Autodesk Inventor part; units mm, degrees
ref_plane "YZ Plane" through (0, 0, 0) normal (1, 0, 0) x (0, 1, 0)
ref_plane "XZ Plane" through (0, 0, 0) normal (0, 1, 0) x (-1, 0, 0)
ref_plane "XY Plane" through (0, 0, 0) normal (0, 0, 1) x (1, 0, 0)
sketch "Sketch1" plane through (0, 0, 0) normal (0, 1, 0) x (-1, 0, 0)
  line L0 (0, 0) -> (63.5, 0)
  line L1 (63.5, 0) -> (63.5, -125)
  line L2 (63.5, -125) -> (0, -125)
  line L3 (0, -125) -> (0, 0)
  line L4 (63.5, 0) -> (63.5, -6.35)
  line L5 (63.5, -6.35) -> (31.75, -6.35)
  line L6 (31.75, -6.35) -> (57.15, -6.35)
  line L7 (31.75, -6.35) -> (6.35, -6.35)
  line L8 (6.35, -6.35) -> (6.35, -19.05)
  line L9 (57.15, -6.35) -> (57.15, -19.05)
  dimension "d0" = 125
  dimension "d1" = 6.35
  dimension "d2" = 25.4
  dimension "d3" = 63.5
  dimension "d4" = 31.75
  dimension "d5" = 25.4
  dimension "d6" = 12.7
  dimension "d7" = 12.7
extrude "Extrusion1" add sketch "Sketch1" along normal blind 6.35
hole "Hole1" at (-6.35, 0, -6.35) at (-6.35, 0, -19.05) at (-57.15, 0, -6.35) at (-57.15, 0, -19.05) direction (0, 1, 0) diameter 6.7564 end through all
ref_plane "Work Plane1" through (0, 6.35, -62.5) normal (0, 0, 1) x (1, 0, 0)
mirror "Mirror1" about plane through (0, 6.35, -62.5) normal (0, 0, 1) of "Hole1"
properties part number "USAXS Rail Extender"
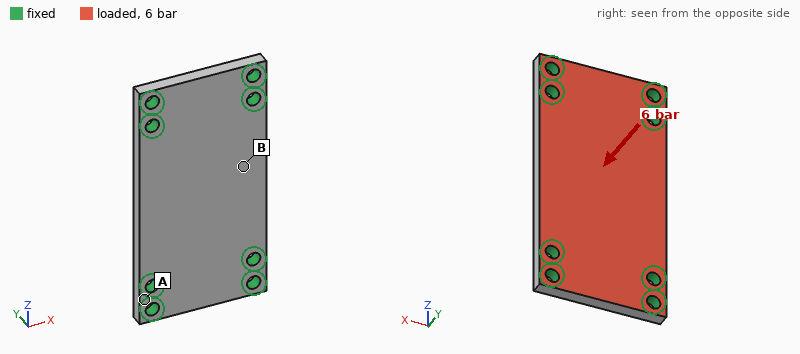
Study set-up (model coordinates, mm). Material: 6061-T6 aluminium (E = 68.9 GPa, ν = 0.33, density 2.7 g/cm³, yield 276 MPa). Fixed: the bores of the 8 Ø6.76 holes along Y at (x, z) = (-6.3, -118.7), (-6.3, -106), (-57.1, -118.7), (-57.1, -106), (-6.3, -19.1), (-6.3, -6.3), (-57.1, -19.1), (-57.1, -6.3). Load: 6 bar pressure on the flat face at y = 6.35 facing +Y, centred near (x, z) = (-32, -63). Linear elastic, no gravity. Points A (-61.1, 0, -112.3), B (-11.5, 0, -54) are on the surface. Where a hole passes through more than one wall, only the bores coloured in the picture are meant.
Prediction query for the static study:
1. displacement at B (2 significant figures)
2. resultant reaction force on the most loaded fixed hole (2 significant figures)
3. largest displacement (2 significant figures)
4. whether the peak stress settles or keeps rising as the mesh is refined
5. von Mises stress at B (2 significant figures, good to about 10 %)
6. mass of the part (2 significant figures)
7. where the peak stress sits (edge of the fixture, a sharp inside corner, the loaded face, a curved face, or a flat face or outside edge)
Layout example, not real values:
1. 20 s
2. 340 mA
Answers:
1. 63 µm
2. 1.1 kN
3. 70 µm
4. keeps rising
5. 25 MPa
6. 130 g
7. edge of the fixture
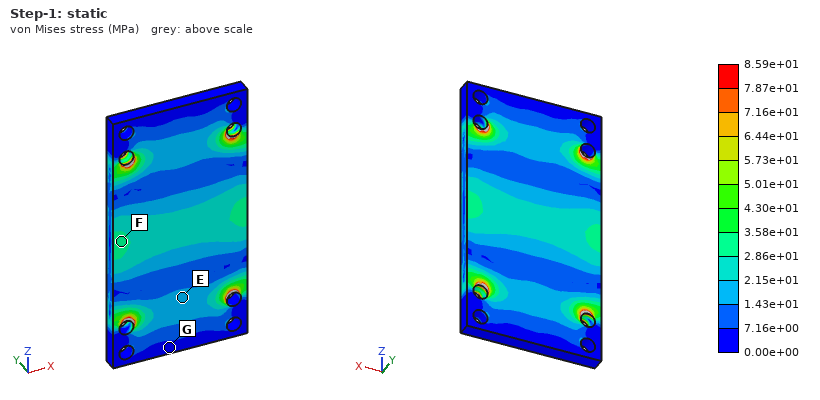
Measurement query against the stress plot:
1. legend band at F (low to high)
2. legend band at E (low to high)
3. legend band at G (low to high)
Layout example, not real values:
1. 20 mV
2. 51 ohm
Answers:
1. 2.86e+01 to 3.58e+01 MPa
2. 1.43e+01 to 2.15e+01 MPa
3. 0.00e+00 to 7.16e+00 MPa
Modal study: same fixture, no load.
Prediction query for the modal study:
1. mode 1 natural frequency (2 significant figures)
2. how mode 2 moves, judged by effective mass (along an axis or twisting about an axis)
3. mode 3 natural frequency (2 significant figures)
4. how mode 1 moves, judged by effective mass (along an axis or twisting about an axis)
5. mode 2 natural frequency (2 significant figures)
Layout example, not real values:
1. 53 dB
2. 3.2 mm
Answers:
1. 4100 Hz
2. twisting about Z
3. 10 kHz
4. along Y
5. 6000 Hz
